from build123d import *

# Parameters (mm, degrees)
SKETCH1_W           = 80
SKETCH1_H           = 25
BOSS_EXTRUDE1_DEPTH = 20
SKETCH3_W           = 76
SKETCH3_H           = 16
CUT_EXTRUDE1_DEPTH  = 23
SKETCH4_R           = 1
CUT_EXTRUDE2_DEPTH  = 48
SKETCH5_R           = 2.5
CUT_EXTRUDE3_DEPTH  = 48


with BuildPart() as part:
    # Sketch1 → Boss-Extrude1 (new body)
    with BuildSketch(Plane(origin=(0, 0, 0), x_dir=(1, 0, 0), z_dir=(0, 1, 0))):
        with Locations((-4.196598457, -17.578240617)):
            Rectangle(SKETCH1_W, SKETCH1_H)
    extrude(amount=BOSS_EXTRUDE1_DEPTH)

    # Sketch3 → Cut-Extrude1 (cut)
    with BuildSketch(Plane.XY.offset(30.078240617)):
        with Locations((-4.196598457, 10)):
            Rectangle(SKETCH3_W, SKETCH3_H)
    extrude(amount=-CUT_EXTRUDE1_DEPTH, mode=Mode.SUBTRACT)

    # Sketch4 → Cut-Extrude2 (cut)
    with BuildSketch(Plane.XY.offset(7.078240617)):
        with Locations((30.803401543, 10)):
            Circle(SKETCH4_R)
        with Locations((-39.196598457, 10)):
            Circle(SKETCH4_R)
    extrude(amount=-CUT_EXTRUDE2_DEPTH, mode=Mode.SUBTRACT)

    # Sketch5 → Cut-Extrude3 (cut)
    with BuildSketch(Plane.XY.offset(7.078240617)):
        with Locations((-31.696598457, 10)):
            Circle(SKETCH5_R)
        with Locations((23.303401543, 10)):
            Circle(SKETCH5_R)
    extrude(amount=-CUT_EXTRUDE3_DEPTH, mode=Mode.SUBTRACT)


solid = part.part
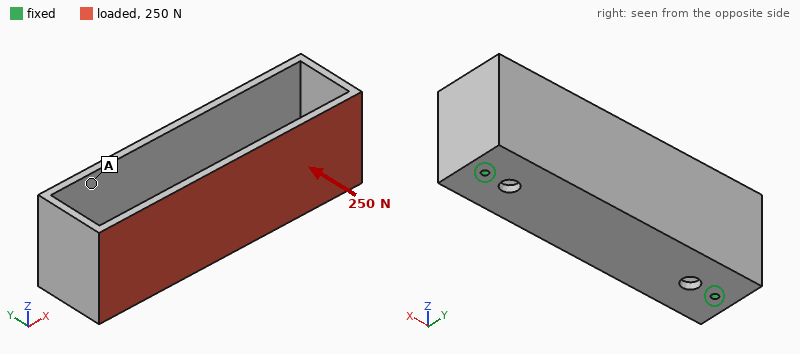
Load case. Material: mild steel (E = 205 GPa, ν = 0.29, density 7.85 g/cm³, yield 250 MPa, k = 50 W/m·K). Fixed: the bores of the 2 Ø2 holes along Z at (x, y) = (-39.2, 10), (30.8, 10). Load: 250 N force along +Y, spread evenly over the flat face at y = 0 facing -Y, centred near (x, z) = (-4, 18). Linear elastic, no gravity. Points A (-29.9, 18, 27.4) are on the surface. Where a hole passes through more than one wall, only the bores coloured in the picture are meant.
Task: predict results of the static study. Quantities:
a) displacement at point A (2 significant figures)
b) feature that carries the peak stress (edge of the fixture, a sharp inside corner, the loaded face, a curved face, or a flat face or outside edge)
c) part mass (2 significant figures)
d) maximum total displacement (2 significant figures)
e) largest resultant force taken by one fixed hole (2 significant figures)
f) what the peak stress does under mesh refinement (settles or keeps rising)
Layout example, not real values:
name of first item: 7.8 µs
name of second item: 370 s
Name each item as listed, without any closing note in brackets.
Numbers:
displacement at point A: 30 µm
feature that carries the peak stress: edge of the fixture
part mass: 94 g
maximum total displacement: 73 µm
largest resultant force taken by one fixed hole: 130 N
what the peak stress does under mesh refinement: keeps rising
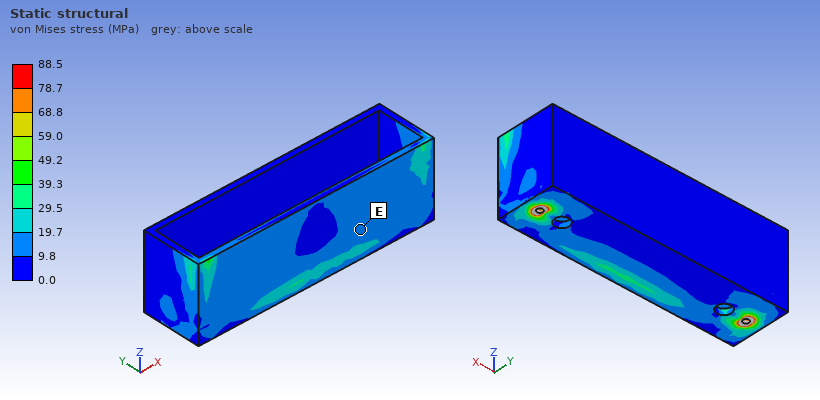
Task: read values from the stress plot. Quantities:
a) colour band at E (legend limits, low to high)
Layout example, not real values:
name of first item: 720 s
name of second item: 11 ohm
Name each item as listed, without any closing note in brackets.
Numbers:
colour band at E: 9.8 to 19.7 MPa
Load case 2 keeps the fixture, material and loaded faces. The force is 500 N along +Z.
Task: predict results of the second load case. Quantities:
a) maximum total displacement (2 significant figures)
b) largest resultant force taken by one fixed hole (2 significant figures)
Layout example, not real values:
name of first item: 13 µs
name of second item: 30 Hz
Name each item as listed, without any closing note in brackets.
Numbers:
maximum total displacement: 75 µm
largest resultant force taken by one fixed hole: 260 N
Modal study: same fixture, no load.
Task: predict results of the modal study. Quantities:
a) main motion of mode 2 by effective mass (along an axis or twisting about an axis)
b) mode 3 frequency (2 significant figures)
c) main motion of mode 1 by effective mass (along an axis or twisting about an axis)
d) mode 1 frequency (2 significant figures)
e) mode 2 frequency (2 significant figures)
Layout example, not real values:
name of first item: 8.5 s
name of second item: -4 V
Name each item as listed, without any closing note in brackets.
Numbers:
main motion of mode 2 by effective mass: twisting about Z
mode 3 frequency: 3100 Hz
main motion of mode 1 by effective mass: along Y
mode 1 frequency: 1500 Hz
mode 2 frequency: 2600 Hz
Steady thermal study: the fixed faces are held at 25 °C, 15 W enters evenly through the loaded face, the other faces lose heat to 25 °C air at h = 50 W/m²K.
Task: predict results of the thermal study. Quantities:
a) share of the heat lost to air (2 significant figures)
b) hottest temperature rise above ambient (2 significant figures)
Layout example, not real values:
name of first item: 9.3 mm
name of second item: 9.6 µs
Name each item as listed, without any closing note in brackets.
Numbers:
share of the heat lost to air: 55 %
hottest temperature rise above ambient: 37 K
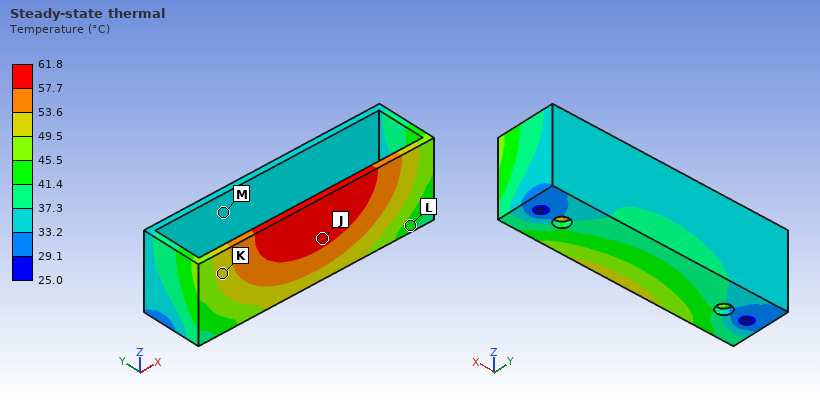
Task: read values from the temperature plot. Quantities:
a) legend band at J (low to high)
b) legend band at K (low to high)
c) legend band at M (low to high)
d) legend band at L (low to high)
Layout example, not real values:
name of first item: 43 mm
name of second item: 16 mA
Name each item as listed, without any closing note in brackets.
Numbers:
legend band at J: 57.7 to 61.8 °C
legend band at K: 49.5 to 53.6 °C
legend band at M: 33.2 to 37.3 °C
legend band at L: 41.4 to 45.5 °C
